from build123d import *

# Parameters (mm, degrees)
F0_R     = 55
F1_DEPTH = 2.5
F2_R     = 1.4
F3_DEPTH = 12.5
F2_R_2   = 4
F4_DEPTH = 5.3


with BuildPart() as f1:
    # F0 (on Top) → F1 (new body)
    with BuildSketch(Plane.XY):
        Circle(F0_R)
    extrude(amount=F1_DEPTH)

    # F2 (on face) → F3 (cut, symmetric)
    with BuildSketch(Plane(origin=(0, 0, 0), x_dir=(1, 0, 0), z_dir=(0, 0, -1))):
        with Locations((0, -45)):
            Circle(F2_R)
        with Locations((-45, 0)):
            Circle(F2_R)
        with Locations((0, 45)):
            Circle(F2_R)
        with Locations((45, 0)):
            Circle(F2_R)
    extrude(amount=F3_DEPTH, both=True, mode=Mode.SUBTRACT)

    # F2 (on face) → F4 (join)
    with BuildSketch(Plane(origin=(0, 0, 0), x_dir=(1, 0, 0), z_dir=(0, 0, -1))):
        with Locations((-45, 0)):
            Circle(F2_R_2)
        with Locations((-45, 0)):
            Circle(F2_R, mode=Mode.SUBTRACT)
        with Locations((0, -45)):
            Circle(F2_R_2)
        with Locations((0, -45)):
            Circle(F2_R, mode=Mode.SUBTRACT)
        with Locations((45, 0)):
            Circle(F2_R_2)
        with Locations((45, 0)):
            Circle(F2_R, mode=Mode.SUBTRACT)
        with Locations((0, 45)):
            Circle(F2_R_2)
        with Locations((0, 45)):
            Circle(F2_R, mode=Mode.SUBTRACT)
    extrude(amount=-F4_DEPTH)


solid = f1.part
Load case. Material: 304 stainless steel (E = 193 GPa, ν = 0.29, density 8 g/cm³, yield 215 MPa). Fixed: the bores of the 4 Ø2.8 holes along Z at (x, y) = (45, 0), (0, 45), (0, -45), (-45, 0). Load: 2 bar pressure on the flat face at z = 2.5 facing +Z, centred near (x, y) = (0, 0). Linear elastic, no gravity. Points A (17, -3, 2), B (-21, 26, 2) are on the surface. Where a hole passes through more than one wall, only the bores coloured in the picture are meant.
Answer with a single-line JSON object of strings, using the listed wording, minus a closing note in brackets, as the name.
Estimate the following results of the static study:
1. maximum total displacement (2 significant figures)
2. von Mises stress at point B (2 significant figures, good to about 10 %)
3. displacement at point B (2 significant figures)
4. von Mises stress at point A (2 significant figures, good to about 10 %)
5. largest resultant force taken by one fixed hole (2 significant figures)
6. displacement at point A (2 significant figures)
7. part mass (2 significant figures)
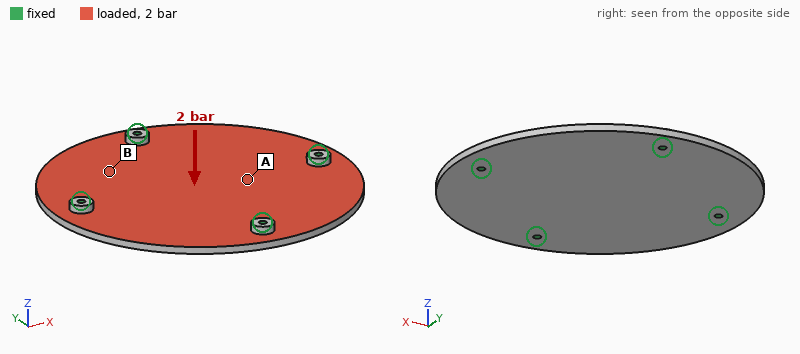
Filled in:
{"maximum total displacement": "66 µm", "von Mises stress at point B": "39 MPa", "displacement at point B": "42 µm", "von Mises stress at point A": "23 MPa", "largest resultant force taken by one fixed hole": "480 N", "displacement at point A": "54 µm", "part mass": "190 g"}
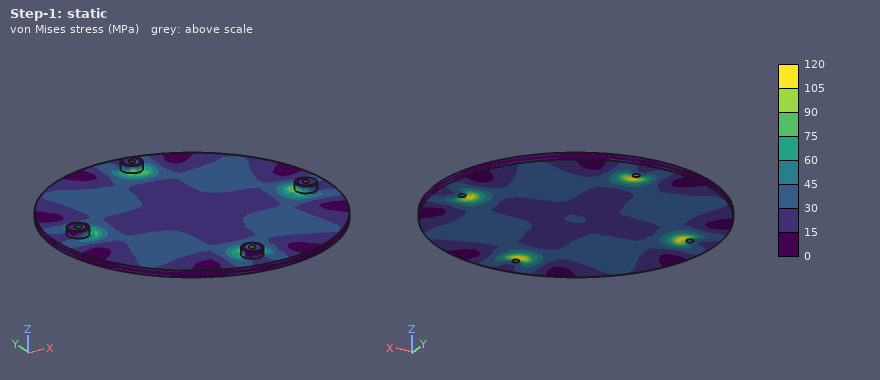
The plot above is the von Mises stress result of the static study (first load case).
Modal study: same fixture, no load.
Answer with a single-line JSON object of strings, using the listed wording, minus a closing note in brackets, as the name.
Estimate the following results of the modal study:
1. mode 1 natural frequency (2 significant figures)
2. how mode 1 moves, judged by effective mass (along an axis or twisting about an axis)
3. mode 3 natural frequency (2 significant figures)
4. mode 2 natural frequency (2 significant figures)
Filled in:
{"mode 1 natural frequency": "2300 Hz", "how mode 1 moves, judged by effective mass": "along Z", "mode 3 natural frequency": "2600 Hz", "mode 2 natural frequency": "2500 Hz"}
